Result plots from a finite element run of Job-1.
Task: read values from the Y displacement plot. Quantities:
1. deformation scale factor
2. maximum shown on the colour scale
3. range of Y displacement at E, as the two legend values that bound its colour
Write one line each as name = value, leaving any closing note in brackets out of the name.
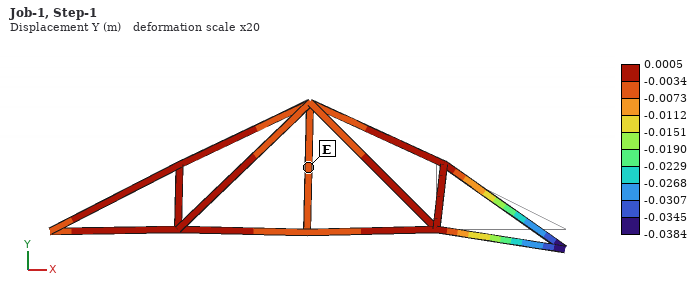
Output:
deformation scale factor = 20
maximum shown on the colour scale = 0.0005 m
range of Y displacement at E, as the two legend values that bound its colour = -0.0073 to -0.0034 m
